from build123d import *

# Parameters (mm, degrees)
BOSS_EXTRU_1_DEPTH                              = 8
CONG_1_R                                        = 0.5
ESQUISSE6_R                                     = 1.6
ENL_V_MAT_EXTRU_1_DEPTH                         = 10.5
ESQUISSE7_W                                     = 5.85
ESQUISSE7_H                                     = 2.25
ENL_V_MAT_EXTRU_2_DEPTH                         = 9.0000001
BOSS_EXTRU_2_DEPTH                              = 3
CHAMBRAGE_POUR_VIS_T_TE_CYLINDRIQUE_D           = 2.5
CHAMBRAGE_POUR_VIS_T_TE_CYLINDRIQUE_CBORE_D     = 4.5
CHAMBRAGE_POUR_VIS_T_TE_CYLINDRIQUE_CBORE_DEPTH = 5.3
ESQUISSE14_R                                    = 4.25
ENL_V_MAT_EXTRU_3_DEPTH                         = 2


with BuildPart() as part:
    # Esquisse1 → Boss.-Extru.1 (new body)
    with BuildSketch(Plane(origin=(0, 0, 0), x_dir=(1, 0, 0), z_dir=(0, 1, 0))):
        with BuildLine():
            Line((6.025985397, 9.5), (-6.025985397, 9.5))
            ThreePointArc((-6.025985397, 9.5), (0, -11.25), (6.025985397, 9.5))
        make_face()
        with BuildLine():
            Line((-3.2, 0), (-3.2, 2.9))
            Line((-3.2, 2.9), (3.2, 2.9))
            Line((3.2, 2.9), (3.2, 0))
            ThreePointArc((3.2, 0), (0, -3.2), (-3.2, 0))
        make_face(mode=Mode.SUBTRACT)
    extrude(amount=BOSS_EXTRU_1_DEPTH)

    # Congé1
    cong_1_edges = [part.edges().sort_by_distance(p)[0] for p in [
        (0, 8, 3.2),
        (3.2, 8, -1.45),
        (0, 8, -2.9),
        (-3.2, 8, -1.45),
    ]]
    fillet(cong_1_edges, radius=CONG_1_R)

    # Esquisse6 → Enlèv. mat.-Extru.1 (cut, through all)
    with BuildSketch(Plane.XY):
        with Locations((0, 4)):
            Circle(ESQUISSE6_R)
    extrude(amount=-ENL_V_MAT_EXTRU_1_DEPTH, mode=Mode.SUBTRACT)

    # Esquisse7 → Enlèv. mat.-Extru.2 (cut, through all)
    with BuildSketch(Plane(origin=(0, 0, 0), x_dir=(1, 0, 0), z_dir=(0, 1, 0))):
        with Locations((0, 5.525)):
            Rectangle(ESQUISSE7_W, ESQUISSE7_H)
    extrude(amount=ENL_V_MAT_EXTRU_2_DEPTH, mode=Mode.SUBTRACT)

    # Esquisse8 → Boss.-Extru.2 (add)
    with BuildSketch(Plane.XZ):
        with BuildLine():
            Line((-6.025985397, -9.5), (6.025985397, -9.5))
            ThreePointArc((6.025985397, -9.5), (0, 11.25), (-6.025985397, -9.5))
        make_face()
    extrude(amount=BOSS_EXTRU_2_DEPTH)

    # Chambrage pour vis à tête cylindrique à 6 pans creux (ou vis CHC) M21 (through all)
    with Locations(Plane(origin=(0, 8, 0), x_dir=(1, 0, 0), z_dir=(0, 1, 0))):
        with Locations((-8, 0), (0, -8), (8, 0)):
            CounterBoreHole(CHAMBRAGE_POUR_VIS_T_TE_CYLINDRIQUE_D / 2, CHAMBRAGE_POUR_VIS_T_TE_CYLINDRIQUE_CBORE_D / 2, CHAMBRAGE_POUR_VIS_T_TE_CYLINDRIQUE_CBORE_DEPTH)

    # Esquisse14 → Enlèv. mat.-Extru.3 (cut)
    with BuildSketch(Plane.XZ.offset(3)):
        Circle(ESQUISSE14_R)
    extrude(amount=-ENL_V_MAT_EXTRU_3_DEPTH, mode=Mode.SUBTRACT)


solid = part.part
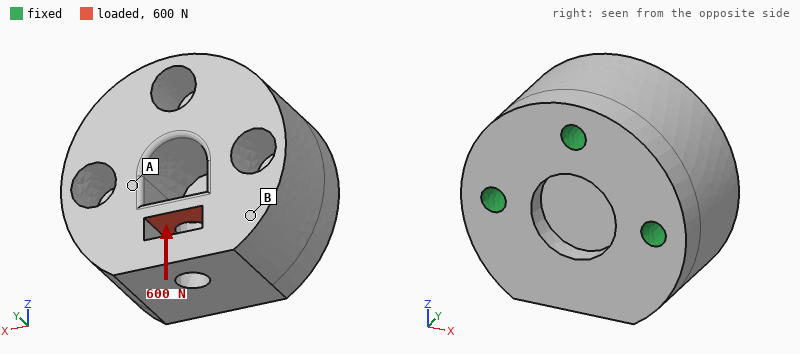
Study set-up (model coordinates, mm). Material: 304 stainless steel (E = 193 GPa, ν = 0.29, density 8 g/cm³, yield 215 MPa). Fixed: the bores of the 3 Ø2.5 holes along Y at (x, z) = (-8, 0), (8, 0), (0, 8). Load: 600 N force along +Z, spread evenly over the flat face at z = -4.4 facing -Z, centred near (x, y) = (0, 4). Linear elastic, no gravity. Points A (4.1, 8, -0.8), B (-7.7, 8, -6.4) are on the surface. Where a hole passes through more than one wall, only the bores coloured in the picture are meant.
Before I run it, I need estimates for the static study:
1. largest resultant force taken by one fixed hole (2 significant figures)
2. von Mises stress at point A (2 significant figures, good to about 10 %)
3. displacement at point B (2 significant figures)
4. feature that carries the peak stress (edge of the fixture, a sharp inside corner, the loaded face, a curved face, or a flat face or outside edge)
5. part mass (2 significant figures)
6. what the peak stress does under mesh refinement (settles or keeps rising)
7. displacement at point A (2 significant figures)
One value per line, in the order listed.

240 N
15 MPa
0.74 µm
a sharp inside corner
27 g
keeps rising
0.68 µm
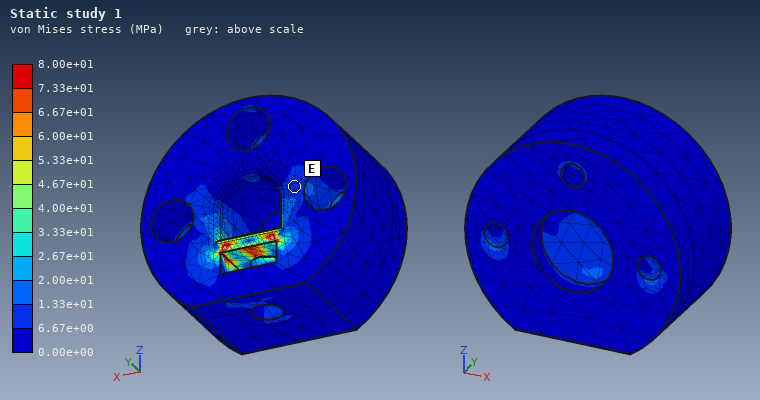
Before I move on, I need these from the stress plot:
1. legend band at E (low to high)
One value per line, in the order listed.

6.67e+00 to 1.33e+01 MPa
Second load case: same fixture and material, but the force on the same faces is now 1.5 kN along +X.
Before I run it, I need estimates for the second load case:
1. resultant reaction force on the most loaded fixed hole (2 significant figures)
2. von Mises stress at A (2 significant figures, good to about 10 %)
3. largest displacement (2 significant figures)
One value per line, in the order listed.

860 N
22 MPa
2.7 µm
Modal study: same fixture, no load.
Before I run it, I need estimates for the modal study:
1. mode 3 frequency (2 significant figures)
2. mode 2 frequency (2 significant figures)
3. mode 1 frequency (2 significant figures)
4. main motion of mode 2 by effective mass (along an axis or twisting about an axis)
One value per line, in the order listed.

54 kHz
49 kHz
33 kHz
along X
